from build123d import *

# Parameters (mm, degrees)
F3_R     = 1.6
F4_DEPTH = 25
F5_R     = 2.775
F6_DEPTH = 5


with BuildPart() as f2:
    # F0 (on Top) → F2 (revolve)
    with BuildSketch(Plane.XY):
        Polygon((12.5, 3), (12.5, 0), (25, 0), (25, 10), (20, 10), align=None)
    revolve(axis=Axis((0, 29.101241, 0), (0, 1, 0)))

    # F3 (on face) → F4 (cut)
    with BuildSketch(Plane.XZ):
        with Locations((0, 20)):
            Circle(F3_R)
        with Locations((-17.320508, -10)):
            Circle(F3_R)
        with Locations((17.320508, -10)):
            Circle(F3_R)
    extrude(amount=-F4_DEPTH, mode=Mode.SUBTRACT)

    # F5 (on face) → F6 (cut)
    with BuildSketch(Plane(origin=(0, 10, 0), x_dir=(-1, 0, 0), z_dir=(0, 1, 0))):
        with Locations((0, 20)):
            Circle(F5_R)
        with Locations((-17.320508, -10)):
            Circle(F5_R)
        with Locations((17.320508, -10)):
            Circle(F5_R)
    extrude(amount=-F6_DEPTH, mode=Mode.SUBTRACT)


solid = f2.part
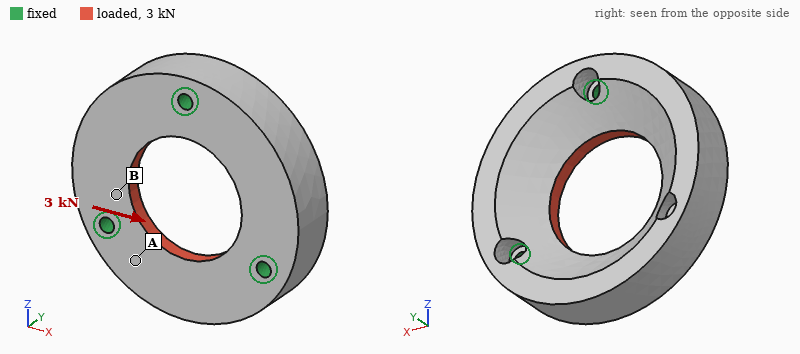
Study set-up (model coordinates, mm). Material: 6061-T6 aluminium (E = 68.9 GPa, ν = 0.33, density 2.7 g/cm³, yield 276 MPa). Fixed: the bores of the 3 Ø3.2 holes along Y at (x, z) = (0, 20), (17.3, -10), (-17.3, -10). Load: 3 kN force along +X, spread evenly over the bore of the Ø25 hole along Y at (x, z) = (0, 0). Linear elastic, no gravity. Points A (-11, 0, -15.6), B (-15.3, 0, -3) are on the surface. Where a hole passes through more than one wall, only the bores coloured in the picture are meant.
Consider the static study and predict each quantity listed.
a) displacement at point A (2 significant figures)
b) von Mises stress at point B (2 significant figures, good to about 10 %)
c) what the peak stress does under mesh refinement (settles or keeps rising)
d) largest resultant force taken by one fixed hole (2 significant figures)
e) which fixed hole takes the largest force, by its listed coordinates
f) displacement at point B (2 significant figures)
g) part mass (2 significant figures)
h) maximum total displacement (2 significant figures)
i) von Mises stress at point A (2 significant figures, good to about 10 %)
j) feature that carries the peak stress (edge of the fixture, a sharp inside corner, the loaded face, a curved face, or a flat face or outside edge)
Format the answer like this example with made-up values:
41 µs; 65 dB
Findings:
1.3 µm; 17 MPa; keeps rising; 1.2 kN; (0, 20); 3.1 µm; 32 g; 6.1 µm; 5.9 MPa; edge of the fixture
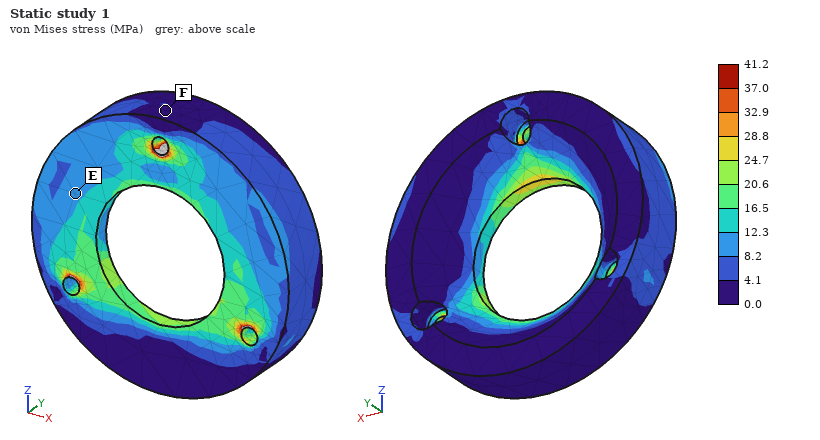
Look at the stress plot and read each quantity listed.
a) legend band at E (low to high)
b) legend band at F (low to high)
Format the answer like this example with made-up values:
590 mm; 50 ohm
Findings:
8.2 to 12.3 MPa; 0.0 to 4.1 MPa
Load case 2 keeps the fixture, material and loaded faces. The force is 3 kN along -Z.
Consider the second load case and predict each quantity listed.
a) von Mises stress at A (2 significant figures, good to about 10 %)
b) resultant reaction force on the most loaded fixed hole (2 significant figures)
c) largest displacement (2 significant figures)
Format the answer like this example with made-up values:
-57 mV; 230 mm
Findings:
15 MPa; 1.1 kN; 6.9 µm
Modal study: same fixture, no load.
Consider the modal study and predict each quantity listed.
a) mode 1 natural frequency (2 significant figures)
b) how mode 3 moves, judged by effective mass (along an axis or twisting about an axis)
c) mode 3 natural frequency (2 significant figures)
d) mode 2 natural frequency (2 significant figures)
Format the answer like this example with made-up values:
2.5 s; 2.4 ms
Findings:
12 kHz; along Y; 15 kHz; 12 kHz
